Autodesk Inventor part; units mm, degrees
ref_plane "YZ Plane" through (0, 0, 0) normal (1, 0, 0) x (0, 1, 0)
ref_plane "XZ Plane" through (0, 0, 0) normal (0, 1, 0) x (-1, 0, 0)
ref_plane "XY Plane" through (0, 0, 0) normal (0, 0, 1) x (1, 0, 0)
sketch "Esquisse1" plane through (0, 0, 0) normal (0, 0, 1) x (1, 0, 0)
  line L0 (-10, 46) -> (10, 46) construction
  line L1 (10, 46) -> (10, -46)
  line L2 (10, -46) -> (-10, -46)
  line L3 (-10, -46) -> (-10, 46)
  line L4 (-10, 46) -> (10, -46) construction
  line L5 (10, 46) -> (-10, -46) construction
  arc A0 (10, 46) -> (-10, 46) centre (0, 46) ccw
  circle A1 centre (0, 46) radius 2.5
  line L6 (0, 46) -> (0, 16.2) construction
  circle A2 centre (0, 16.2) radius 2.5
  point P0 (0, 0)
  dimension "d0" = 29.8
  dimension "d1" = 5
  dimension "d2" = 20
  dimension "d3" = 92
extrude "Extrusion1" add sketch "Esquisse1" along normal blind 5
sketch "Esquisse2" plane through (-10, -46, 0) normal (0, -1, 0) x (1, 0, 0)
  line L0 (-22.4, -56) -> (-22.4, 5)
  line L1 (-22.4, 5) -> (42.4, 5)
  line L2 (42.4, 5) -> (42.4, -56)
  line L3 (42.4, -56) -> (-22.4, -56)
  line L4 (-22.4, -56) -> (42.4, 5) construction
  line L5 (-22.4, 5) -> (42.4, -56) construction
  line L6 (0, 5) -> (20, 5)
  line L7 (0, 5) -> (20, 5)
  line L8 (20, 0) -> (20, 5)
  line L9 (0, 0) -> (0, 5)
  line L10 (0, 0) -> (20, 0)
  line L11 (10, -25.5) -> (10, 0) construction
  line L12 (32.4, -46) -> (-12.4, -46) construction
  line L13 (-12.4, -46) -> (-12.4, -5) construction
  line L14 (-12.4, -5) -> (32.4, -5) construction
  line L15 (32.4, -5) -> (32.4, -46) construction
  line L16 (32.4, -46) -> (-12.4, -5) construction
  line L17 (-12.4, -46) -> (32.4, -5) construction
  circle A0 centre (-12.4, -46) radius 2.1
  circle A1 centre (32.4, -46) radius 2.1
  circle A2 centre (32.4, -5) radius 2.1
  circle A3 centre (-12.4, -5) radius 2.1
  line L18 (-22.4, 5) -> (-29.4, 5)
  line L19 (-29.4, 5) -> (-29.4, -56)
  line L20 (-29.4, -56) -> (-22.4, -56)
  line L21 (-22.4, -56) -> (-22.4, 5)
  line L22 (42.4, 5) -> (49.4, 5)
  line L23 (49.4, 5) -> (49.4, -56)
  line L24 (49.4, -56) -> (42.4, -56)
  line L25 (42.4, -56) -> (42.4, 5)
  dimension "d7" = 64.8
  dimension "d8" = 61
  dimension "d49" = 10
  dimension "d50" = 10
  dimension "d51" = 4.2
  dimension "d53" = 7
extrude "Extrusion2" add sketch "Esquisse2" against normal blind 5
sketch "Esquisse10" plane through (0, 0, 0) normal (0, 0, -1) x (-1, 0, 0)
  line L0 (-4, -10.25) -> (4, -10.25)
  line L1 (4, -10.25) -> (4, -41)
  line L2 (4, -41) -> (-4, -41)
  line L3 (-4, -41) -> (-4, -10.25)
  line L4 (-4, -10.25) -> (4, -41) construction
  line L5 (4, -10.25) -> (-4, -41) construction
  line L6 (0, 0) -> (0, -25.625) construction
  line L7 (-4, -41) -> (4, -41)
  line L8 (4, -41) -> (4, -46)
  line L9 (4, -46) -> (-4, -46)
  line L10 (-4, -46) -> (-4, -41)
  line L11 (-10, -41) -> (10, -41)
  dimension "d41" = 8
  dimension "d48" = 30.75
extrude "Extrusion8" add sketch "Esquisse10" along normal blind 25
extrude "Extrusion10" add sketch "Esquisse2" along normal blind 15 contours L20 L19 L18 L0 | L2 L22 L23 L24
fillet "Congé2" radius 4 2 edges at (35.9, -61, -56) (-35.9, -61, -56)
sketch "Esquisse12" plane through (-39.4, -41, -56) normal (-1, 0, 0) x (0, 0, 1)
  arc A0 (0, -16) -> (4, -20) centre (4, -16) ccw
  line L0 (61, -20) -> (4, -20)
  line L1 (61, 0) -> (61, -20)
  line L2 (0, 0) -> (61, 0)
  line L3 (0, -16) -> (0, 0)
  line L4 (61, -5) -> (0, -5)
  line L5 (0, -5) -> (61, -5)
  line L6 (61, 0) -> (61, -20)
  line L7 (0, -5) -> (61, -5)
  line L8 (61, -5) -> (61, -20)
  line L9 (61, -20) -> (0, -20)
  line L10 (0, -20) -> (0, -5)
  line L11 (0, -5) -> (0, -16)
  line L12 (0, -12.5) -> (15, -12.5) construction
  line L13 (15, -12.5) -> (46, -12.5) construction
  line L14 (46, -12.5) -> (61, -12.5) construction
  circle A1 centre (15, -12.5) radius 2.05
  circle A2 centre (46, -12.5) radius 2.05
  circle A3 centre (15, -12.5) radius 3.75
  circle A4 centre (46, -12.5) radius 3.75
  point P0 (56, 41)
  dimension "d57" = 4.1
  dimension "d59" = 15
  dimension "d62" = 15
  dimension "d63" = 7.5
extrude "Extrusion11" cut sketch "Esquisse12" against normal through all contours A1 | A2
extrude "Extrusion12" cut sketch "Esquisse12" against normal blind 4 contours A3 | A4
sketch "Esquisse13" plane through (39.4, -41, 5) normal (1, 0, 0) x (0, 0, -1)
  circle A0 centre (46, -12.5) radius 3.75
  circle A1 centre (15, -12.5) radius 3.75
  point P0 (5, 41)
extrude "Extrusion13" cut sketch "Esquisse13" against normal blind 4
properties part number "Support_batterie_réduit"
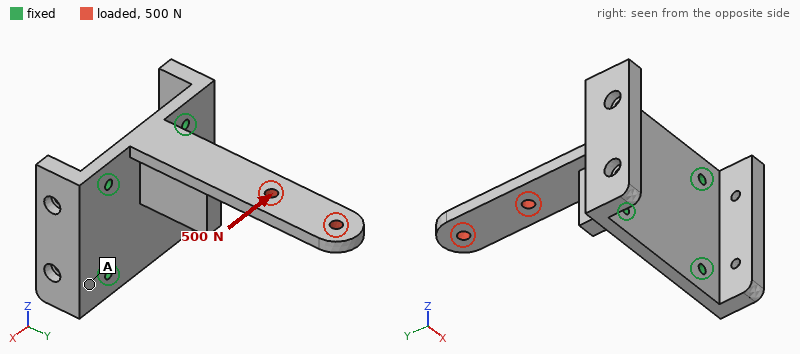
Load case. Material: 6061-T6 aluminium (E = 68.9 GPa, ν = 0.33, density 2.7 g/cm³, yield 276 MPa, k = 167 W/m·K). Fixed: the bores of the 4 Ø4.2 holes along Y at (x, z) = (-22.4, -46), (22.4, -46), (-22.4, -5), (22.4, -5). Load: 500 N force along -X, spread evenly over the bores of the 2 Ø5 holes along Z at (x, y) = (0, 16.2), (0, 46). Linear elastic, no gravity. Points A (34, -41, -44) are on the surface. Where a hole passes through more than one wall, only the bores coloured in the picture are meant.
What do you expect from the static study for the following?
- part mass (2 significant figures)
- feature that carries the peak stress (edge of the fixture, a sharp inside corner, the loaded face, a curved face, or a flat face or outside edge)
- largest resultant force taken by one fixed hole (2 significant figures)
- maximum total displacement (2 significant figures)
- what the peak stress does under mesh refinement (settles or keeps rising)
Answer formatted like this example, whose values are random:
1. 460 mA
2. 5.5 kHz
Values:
1. 140 g
2. edge of the fixture
3. 1.1 kN
4. 0.66 mm
5. keeps rising
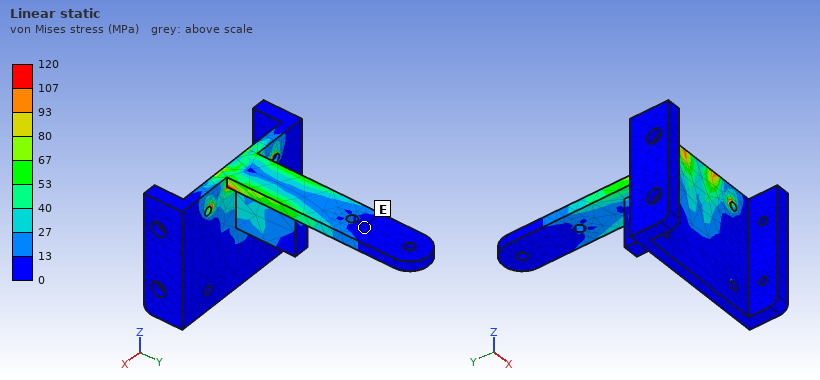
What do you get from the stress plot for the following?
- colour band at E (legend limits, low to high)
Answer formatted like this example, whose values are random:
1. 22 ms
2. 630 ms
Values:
1. 0 to 13 MPa
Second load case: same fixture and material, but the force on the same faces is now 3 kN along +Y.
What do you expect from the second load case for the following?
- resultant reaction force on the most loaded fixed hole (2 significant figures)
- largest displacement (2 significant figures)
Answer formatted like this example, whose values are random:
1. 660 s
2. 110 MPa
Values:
1. 1.8 kN
2. 0.37 mm
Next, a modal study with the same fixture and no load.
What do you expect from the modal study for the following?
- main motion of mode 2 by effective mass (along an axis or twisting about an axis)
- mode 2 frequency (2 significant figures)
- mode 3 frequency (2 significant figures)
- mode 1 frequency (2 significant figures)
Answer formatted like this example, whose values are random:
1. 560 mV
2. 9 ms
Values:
1. along X
2. 1400 Hz
3. 3300 Hz
4. 830 Hz
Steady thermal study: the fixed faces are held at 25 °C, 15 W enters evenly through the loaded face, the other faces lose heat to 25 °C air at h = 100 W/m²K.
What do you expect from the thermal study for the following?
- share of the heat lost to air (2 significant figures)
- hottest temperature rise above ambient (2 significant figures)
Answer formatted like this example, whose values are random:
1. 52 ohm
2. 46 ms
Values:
1. 62 %
2. 32 K
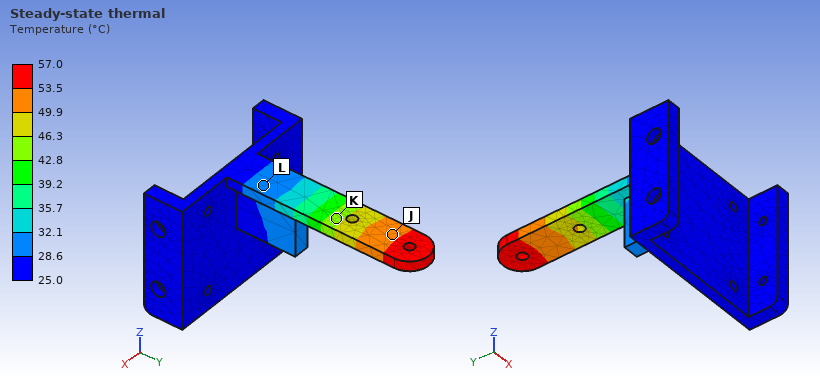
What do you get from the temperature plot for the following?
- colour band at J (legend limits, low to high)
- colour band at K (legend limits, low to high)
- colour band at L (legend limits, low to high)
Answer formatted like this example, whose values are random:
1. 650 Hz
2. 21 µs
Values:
1. 49.9 to 53.5 °C
2. 42.8 to 46.3 °C
3. 28.6 to 32.1 °C
